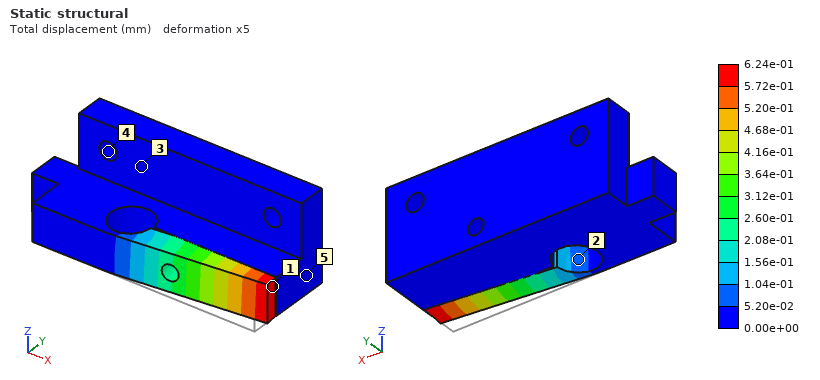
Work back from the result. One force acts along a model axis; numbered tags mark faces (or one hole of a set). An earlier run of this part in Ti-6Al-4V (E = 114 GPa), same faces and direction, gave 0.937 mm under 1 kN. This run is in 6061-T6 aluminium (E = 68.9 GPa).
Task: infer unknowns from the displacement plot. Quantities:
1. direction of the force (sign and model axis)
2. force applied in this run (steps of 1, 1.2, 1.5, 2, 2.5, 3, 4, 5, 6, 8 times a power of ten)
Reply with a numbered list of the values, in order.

1. +Y
2. 400 N
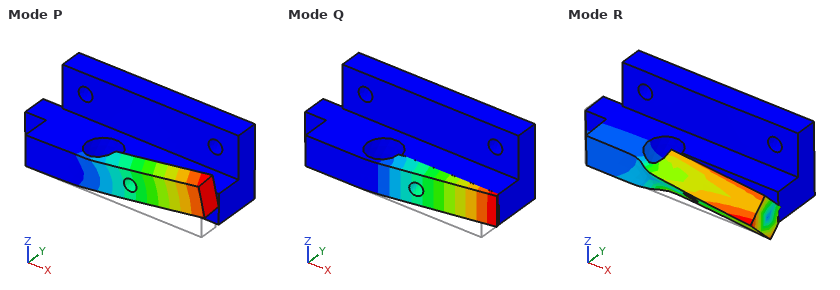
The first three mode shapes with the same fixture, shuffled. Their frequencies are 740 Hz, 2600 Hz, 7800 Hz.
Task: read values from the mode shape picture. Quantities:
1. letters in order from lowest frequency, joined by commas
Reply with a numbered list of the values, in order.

1. Q, P, R
